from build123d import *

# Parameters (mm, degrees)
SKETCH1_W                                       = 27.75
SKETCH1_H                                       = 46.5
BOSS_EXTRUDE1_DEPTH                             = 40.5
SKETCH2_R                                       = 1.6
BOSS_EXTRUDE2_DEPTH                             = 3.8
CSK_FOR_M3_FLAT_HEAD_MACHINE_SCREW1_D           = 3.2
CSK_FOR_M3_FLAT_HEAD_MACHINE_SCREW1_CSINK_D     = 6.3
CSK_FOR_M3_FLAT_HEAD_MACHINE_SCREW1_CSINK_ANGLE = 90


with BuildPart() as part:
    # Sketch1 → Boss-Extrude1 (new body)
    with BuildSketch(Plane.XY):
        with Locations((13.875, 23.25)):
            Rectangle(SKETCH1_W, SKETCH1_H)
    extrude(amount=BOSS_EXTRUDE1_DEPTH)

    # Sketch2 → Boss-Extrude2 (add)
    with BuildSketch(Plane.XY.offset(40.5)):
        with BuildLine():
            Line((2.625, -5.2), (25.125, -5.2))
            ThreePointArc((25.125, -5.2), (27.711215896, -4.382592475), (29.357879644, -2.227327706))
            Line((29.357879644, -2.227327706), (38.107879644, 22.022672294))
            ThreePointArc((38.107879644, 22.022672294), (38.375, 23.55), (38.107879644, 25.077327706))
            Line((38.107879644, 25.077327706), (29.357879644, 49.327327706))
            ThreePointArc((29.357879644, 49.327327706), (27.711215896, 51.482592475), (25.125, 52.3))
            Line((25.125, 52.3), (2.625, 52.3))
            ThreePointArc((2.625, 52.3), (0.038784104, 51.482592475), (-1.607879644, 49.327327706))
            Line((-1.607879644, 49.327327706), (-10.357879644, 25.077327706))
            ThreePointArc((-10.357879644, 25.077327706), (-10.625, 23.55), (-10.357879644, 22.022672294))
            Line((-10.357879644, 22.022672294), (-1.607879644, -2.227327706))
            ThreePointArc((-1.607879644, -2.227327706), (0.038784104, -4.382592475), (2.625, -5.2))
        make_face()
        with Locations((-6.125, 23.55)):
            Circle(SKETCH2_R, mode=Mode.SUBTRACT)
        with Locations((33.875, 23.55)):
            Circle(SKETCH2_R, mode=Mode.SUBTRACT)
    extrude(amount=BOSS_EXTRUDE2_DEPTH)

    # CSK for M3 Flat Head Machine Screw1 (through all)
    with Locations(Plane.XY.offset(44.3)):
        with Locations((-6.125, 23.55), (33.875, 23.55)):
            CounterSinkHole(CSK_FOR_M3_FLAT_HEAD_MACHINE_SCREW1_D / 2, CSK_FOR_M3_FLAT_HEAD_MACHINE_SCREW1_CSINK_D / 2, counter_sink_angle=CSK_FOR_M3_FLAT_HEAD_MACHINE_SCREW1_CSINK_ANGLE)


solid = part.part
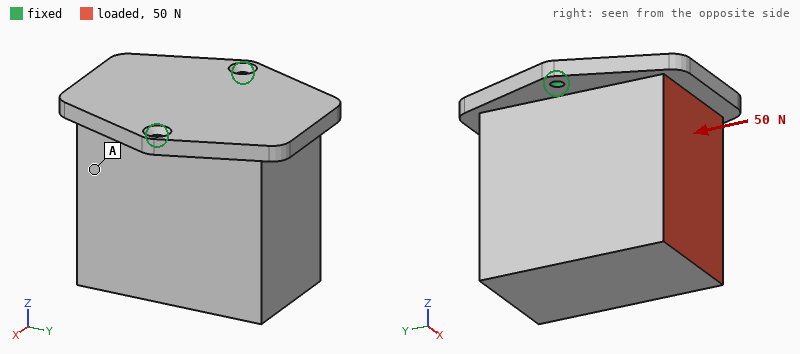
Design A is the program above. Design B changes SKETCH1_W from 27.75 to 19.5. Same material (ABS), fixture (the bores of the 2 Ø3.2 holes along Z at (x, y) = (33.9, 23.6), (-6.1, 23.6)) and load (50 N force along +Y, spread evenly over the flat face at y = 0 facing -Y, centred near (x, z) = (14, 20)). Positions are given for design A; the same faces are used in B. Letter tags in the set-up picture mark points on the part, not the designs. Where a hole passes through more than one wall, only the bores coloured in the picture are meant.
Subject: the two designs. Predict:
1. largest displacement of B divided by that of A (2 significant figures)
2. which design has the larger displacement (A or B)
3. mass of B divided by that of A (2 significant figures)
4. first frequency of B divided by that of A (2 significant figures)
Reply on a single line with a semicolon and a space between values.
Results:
1.2; B; 0.74; 1.1
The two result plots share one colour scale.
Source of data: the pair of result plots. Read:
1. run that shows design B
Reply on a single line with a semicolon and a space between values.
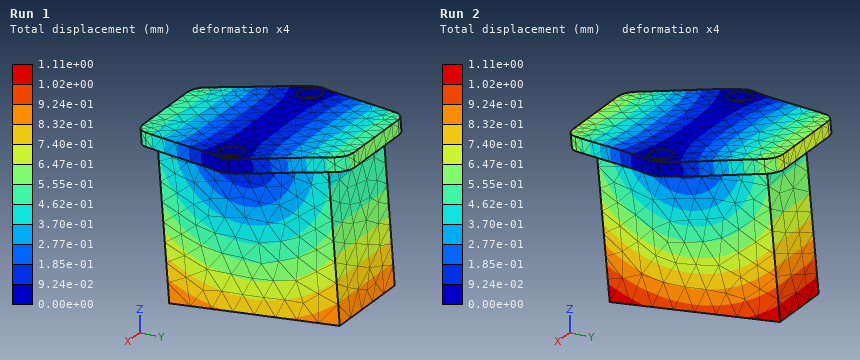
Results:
Run 2
